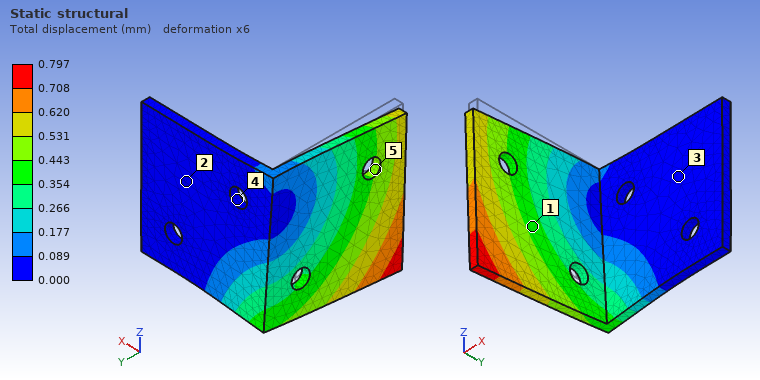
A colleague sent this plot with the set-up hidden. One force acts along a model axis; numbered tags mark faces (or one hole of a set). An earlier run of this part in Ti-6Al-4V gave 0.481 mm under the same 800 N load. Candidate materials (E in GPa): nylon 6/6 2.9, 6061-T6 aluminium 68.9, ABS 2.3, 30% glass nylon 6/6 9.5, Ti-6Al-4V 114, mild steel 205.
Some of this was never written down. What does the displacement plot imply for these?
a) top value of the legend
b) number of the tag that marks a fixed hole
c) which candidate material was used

0.797 mm
4
6061-T6 aluminium
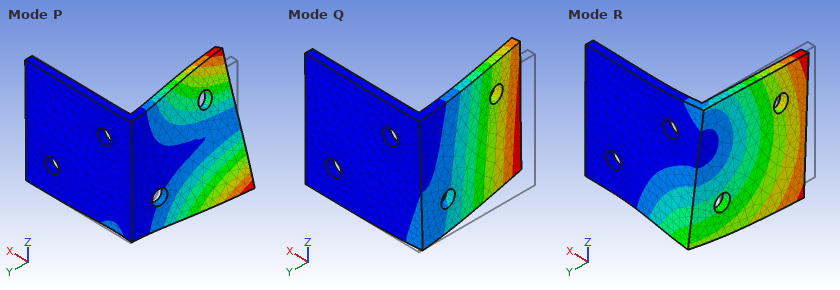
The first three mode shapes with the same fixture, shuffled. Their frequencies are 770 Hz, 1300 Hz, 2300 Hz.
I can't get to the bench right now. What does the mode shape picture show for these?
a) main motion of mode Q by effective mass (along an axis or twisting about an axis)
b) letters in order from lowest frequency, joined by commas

along X
Q, R, P
